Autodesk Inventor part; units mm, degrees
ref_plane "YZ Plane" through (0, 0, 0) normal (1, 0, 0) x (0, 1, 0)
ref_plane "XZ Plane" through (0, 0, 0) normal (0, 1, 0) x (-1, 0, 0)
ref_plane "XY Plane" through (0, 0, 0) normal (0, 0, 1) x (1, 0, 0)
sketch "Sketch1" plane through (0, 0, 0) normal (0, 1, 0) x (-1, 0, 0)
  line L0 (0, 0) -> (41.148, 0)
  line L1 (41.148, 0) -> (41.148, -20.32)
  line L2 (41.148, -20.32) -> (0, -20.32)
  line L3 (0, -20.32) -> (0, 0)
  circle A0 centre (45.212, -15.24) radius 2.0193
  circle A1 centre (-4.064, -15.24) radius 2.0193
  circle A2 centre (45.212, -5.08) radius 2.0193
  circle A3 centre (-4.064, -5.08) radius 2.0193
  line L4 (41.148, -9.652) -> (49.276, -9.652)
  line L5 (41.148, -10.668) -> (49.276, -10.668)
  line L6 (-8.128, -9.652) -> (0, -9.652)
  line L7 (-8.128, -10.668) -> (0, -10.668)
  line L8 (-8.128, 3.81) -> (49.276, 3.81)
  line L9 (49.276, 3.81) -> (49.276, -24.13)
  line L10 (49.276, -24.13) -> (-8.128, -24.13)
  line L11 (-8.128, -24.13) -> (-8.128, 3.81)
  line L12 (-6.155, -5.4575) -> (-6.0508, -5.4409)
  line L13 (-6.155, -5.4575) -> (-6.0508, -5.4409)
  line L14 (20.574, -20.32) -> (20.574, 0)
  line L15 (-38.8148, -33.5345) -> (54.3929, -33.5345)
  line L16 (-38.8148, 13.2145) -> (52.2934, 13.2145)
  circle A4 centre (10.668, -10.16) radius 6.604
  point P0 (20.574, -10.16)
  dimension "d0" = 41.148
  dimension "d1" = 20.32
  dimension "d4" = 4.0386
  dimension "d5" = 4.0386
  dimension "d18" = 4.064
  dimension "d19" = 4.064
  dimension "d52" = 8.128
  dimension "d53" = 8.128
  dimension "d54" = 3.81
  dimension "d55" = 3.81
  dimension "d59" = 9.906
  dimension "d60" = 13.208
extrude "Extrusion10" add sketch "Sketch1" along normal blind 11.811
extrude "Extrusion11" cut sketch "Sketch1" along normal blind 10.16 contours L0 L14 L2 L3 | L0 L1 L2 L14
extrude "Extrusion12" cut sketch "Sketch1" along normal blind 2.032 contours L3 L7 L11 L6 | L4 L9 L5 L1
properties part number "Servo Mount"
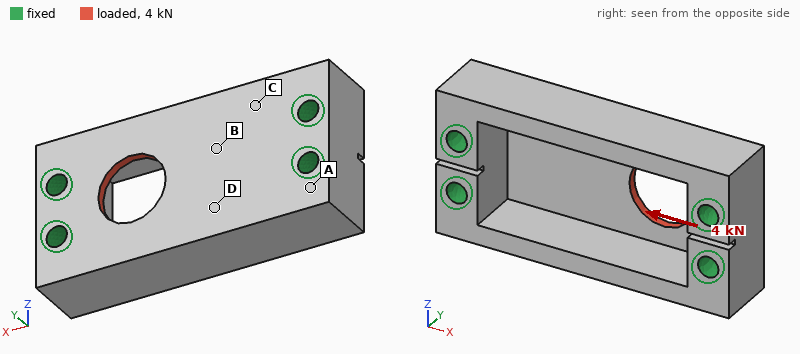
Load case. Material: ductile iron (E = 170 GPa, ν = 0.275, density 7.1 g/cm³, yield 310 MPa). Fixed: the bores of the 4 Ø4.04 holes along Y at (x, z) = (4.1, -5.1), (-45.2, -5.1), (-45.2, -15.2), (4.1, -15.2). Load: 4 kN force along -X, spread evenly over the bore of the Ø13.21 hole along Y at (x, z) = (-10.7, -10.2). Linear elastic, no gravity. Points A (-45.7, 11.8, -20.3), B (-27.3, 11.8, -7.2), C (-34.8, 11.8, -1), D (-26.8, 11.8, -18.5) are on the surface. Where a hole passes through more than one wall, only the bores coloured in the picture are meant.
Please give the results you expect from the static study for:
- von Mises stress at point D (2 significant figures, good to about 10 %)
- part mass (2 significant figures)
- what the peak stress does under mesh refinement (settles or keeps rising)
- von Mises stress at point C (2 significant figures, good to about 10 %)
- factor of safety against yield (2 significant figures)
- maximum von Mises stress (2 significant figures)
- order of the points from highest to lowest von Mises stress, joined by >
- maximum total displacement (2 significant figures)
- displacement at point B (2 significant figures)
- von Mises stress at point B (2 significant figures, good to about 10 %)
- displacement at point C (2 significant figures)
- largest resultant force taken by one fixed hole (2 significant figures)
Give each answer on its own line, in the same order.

30 MPa
68 g
settles
18 MPa
3.0
100 MPa
B > D > C > A
5.8 µm
2.8 µm
42 MPa
1.4 µm
1.3 kN
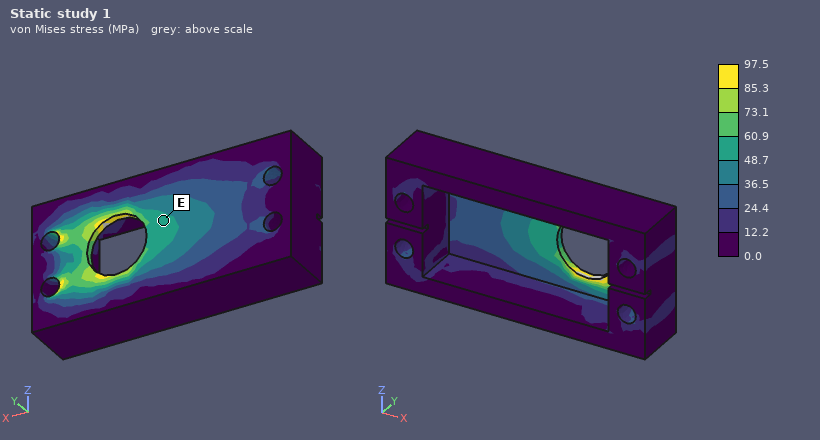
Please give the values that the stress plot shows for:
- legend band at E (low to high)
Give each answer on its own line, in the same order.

48.7 to 60.9 MPa
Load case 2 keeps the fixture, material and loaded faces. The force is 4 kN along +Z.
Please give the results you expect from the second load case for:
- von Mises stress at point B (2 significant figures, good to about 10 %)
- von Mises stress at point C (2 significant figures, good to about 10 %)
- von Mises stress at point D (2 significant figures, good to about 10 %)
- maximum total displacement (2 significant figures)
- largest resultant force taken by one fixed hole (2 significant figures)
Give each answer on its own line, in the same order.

48 MPa
50 MPa
61 MPa
18 µm
1.3 kN
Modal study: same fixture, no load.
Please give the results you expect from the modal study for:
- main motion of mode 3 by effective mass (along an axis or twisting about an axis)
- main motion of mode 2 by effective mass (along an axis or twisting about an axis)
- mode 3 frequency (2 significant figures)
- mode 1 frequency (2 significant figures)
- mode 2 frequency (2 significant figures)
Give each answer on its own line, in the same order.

along Y
along Z
16 kHz
13 kHz
13 kHz
